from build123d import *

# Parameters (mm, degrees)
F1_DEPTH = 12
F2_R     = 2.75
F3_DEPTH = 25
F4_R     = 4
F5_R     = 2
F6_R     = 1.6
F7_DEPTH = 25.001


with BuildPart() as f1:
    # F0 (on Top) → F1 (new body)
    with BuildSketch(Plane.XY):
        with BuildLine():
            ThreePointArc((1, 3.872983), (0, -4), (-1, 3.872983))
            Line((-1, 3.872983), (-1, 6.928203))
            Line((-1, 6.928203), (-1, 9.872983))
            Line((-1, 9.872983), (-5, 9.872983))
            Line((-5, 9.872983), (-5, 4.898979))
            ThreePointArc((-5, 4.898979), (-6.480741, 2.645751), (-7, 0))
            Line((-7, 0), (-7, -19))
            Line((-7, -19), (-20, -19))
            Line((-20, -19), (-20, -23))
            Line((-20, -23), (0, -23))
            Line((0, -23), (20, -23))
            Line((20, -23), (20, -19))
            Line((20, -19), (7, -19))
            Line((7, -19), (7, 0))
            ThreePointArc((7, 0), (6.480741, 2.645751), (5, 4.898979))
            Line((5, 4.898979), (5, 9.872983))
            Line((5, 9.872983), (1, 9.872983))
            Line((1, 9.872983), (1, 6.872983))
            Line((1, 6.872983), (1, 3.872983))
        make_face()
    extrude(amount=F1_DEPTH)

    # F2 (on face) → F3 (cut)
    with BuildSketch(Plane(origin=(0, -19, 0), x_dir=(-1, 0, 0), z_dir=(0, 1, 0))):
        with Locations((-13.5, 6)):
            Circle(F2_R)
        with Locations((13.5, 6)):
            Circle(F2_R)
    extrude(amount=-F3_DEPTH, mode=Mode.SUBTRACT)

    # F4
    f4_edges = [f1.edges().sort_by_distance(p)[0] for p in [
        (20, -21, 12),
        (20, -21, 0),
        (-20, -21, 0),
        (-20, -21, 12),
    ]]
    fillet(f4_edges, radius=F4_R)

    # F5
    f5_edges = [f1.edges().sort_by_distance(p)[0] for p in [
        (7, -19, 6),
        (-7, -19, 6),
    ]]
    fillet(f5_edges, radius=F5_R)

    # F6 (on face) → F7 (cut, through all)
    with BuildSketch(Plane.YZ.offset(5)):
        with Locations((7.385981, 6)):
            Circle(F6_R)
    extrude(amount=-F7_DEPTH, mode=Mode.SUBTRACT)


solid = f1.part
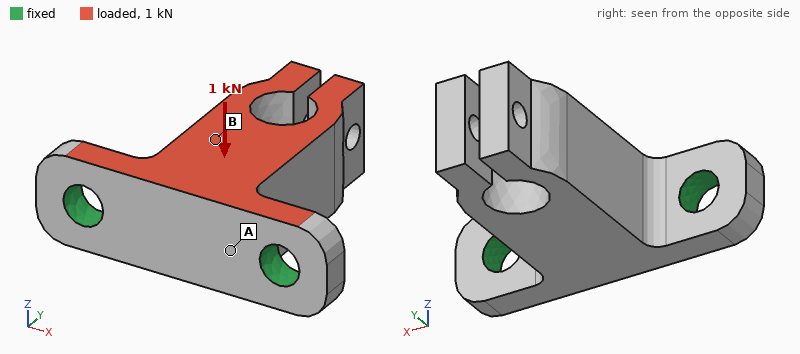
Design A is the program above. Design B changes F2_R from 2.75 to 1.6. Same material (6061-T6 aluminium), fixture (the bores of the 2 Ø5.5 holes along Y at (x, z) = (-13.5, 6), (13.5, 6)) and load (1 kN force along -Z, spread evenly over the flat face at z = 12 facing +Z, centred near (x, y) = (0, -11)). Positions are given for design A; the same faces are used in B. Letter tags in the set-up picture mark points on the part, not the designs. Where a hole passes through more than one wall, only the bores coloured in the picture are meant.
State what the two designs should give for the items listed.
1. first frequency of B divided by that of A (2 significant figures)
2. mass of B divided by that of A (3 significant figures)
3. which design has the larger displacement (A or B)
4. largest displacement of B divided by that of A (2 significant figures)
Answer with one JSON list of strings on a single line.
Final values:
["0.84", "1.02", "B", "1.4"]
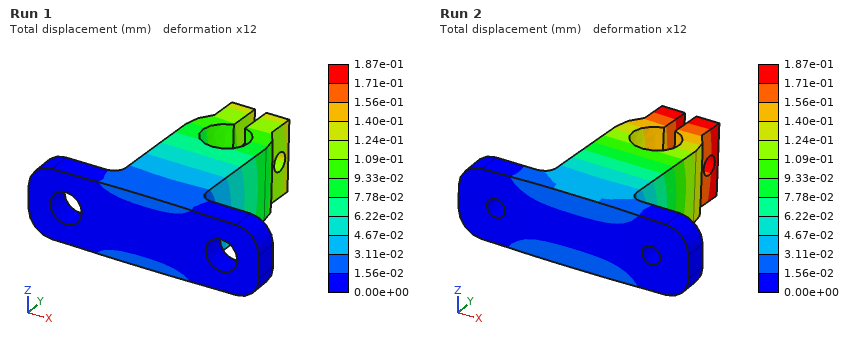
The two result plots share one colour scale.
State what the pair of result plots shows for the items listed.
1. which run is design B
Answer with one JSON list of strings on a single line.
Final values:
["Run 2"]
